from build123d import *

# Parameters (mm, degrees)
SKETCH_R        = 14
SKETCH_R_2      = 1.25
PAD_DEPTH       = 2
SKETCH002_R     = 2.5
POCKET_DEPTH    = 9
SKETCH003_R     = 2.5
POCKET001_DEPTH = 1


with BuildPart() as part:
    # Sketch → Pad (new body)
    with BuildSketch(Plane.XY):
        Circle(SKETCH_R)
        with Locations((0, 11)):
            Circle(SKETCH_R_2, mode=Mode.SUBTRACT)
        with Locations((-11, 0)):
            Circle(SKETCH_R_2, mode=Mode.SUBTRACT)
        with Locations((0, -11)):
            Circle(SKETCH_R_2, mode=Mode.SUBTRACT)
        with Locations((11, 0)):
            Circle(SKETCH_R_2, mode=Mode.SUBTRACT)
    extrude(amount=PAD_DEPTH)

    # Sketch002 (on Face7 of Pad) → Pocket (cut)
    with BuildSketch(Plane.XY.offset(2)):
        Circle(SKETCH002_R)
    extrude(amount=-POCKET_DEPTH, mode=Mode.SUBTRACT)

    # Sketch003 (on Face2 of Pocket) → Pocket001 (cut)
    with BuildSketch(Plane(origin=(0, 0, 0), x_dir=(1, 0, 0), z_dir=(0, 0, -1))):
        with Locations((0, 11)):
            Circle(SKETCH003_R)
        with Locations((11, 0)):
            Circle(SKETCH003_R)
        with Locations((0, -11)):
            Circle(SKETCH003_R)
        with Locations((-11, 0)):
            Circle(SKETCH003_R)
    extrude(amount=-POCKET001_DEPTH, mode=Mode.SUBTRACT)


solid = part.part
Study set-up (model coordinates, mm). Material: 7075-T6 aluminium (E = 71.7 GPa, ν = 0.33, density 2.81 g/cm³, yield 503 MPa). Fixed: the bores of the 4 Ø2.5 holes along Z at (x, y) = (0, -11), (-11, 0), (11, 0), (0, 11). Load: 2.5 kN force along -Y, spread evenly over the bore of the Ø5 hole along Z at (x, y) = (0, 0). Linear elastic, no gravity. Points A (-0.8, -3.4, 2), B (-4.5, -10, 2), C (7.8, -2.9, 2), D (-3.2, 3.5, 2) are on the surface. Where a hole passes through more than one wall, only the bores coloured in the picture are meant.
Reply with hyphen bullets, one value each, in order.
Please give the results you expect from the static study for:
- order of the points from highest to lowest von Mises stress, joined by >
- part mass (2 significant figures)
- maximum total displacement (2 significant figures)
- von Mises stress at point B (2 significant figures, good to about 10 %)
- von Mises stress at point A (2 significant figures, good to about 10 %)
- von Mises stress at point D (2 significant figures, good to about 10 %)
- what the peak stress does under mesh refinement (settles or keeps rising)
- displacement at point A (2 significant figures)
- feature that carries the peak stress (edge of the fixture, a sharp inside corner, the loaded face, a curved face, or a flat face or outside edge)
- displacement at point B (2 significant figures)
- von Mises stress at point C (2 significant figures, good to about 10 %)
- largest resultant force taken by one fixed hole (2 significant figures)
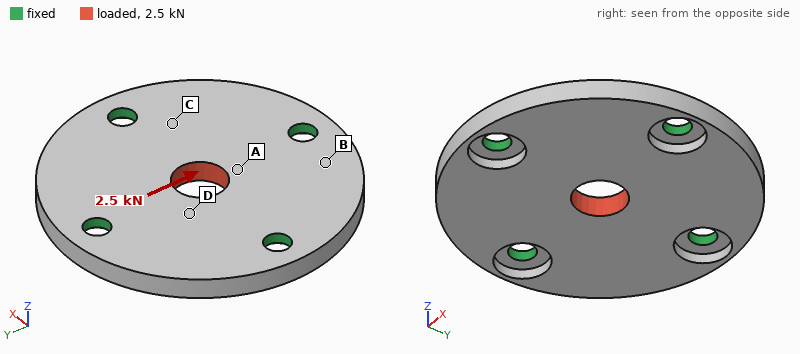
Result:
- A > D > C > B
- 3.1 g
- 11 µm
- 19 MPa
- 82 MPa
- 62 MPa
- keeps rising
- 9.5 µm
- edge of the fixture
- 4.4 µm
- 35 MPa
- 790 N
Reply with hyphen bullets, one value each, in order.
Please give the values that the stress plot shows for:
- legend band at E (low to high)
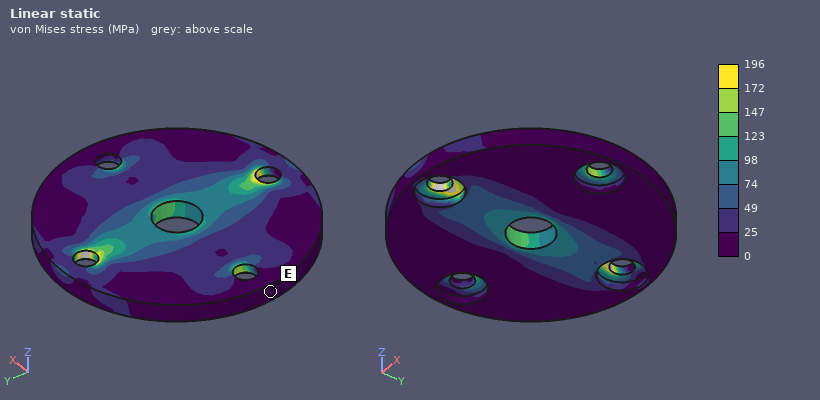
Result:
- 0 to 25 MPa
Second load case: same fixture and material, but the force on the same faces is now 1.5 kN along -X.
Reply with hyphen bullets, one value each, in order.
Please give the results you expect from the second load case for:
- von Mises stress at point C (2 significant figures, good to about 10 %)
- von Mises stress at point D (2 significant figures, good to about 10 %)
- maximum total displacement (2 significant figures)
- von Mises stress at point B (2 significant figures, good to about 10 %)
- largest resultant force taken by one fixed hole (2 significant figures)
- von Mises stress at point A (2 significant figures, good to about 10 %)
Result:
- 32 MPa
- 35 MPa
- 6.8 µm
- 19 MPa
- 480 N
- 41 MPa
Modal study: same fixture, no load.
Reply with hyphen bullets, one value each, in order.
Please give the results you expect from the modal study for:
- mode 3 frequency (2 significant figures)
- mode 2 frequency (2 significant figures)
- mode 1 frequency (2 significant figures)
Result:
- 25 kHz
- 25 kHz
- 23 kHz
